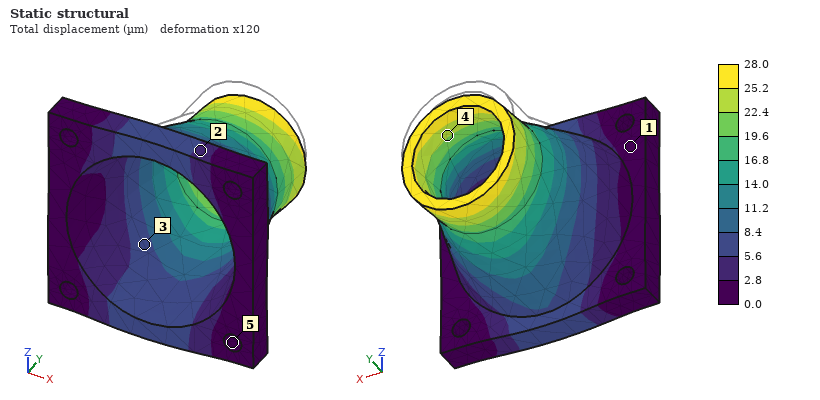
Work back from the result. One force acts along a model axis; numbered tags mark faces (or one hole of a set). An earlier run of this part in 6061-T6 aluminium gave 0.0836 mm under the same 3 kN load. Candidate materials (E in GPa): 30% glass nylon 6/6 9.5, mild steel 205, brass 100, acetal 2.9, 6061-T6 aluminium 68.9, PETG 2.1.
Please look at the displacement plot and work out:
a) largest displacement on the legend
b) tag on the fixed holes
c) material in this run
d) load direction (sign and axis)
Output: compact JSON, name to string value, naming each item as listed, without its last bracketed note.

{"largest displacement on the legend": "28.0 µm", "tag on the fixed holes": "5", "material in this run": "mild steel", "load direction": "-Z"}
